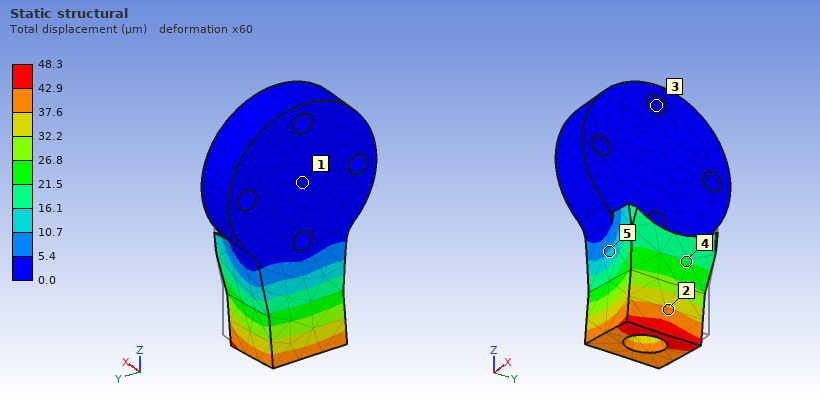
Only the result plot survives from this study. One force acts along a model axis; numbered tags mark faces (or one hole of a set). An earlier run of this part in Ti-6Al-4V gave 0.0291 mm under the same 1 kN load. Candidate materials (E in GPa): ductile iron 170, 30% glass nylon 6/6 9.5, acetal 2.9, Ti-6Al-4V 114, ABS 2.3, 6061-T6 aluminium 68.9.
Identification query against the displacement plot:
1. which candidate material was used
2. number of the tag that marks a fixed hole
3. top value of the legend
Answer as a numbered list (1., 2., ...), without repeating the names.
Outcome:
1. 6061-T6 aluminium
2. 3
3. 48.3 µm
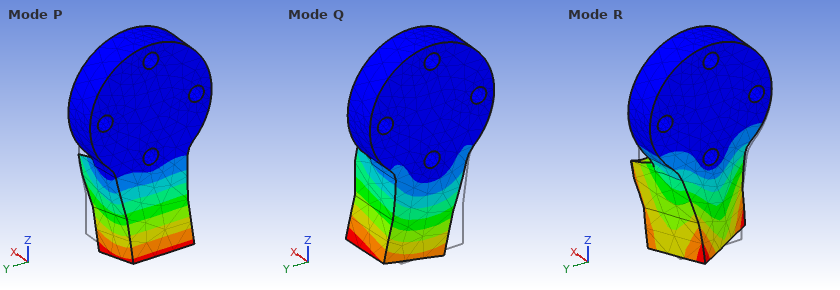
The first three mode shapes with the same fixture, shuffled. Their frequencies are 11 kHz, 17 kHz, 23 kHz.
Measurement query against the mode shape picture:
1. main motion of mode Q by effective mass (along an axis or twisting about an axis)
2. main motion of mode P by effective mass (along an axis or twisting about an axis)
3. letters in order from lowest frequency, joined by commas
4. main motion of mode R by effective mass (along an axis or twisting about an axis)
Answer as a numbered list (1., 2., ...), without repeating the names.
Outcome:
1. along Y
2. along X
3. P, Q, R
4. twisting about Z
